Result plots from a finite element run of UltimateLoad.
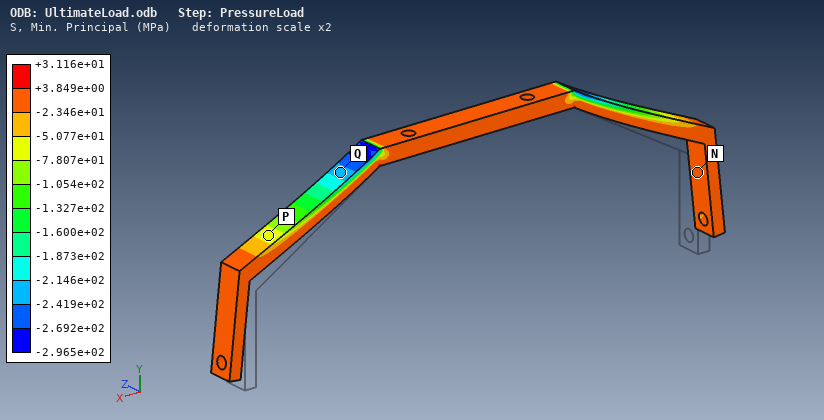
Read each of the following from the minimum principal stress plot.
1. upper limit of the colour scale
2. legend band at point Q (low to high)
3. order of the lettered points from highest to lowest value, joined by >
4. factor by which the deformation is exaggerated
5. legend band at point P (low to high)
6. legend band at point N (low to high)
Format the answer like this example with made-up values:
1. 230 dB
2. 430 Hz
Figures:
1. +3.116e+01 MPa
2. -2.419e+02 to -2.146e+02 MPa
3. N > P > Q
4. 2
5. -7.807e+01 to -5.077e+01 MPa
6. -2.346e+01 to +3.849e+00 MPa
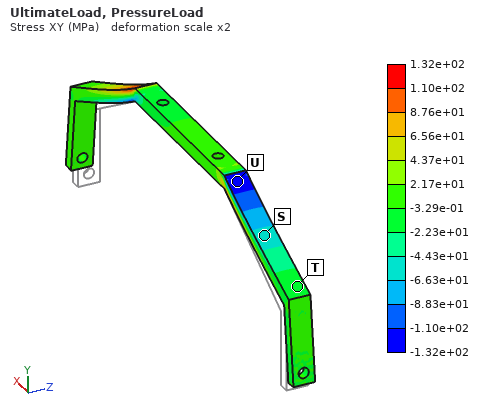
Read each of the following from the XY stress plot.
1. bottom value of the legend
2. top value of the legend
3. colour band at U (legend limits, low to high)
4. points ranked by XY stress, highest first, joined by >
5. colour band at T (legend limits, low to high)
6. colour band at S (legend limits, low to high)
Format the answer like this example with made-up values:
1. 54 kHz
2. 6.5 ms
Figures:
1. -1.32e+02 MPa
2. 1.32e+02 MPa
3. -1.32e+02 to -1.10e+02 MPa
4. T > S > U
5. -2.23e+01 to -3.29e-01 MPa
6. -6.63e+01 to -4.43e+01 MPa
